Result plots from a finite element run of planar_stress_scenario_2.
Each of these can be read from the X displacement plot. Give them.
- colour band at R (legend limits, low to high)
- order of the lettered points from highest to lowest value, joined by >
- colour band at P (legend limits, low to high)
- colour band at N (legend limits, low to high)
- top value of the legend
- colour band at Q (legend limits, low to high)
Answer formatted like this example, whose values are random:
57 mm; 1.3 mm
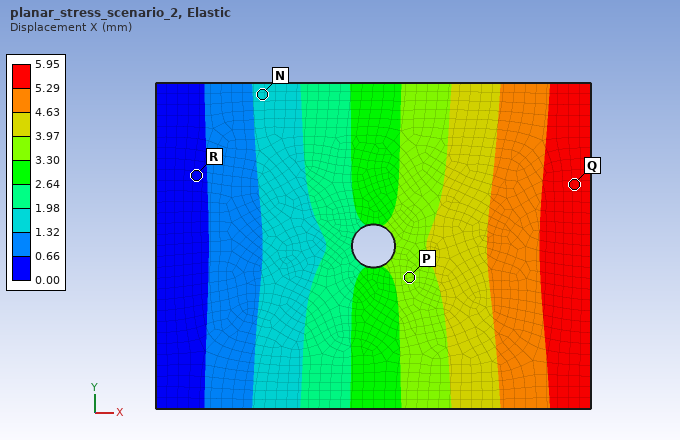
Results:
0.00 to 0.66 mm; Q > P > N > R; 3.30 to 3.97 mm; 1.32 to 1.98 mm; 5.95 mm; 5.29 to 5.95 mm
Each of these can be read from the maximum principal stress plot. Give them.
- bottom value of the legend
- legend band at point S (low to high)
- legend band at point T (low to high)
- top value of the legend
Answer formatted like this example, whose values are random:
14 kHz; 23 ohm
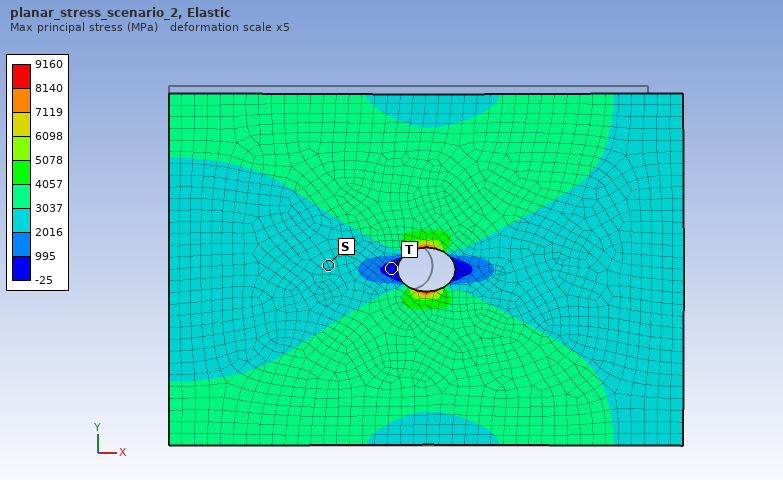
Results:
-25 MPa; 2016 to 3037 MPa; -25 to 995 MPa; 9160 MPa
